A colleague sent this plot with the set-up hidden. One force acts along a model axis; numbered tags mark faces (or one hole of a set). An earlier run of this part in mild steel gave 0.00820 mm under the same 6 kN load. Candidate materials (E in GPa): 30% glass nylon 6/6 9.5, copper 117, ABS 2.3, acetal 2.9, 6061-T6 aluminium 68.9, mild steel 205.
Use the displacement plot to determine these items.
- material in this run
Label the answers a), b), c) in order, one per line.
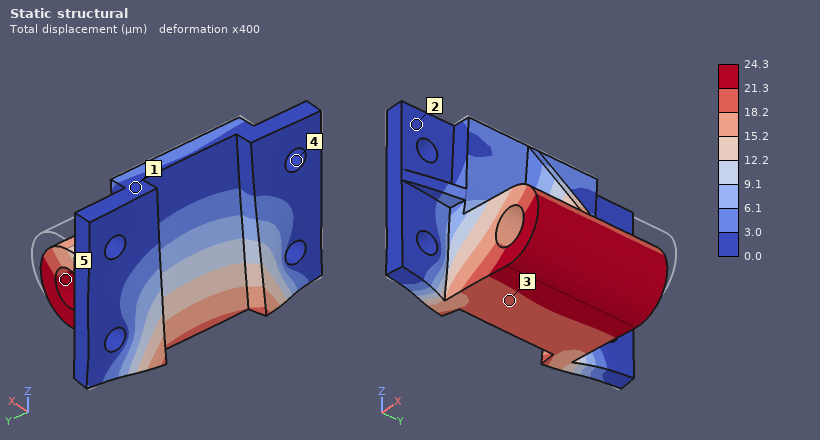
a) 6061-T6 aluminium
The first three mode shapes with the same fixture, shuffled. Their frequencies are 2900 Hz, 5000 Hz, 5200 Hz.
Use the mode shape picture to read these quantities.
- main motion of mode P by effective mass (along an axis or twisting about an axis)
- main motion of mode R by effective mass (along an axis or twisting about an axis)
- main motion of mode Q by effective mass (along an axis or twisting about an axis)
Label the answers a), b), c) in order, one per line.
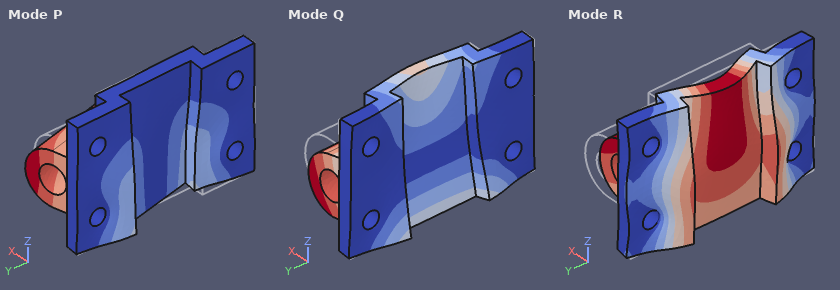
a) along Y
b) along X
c) along Z
